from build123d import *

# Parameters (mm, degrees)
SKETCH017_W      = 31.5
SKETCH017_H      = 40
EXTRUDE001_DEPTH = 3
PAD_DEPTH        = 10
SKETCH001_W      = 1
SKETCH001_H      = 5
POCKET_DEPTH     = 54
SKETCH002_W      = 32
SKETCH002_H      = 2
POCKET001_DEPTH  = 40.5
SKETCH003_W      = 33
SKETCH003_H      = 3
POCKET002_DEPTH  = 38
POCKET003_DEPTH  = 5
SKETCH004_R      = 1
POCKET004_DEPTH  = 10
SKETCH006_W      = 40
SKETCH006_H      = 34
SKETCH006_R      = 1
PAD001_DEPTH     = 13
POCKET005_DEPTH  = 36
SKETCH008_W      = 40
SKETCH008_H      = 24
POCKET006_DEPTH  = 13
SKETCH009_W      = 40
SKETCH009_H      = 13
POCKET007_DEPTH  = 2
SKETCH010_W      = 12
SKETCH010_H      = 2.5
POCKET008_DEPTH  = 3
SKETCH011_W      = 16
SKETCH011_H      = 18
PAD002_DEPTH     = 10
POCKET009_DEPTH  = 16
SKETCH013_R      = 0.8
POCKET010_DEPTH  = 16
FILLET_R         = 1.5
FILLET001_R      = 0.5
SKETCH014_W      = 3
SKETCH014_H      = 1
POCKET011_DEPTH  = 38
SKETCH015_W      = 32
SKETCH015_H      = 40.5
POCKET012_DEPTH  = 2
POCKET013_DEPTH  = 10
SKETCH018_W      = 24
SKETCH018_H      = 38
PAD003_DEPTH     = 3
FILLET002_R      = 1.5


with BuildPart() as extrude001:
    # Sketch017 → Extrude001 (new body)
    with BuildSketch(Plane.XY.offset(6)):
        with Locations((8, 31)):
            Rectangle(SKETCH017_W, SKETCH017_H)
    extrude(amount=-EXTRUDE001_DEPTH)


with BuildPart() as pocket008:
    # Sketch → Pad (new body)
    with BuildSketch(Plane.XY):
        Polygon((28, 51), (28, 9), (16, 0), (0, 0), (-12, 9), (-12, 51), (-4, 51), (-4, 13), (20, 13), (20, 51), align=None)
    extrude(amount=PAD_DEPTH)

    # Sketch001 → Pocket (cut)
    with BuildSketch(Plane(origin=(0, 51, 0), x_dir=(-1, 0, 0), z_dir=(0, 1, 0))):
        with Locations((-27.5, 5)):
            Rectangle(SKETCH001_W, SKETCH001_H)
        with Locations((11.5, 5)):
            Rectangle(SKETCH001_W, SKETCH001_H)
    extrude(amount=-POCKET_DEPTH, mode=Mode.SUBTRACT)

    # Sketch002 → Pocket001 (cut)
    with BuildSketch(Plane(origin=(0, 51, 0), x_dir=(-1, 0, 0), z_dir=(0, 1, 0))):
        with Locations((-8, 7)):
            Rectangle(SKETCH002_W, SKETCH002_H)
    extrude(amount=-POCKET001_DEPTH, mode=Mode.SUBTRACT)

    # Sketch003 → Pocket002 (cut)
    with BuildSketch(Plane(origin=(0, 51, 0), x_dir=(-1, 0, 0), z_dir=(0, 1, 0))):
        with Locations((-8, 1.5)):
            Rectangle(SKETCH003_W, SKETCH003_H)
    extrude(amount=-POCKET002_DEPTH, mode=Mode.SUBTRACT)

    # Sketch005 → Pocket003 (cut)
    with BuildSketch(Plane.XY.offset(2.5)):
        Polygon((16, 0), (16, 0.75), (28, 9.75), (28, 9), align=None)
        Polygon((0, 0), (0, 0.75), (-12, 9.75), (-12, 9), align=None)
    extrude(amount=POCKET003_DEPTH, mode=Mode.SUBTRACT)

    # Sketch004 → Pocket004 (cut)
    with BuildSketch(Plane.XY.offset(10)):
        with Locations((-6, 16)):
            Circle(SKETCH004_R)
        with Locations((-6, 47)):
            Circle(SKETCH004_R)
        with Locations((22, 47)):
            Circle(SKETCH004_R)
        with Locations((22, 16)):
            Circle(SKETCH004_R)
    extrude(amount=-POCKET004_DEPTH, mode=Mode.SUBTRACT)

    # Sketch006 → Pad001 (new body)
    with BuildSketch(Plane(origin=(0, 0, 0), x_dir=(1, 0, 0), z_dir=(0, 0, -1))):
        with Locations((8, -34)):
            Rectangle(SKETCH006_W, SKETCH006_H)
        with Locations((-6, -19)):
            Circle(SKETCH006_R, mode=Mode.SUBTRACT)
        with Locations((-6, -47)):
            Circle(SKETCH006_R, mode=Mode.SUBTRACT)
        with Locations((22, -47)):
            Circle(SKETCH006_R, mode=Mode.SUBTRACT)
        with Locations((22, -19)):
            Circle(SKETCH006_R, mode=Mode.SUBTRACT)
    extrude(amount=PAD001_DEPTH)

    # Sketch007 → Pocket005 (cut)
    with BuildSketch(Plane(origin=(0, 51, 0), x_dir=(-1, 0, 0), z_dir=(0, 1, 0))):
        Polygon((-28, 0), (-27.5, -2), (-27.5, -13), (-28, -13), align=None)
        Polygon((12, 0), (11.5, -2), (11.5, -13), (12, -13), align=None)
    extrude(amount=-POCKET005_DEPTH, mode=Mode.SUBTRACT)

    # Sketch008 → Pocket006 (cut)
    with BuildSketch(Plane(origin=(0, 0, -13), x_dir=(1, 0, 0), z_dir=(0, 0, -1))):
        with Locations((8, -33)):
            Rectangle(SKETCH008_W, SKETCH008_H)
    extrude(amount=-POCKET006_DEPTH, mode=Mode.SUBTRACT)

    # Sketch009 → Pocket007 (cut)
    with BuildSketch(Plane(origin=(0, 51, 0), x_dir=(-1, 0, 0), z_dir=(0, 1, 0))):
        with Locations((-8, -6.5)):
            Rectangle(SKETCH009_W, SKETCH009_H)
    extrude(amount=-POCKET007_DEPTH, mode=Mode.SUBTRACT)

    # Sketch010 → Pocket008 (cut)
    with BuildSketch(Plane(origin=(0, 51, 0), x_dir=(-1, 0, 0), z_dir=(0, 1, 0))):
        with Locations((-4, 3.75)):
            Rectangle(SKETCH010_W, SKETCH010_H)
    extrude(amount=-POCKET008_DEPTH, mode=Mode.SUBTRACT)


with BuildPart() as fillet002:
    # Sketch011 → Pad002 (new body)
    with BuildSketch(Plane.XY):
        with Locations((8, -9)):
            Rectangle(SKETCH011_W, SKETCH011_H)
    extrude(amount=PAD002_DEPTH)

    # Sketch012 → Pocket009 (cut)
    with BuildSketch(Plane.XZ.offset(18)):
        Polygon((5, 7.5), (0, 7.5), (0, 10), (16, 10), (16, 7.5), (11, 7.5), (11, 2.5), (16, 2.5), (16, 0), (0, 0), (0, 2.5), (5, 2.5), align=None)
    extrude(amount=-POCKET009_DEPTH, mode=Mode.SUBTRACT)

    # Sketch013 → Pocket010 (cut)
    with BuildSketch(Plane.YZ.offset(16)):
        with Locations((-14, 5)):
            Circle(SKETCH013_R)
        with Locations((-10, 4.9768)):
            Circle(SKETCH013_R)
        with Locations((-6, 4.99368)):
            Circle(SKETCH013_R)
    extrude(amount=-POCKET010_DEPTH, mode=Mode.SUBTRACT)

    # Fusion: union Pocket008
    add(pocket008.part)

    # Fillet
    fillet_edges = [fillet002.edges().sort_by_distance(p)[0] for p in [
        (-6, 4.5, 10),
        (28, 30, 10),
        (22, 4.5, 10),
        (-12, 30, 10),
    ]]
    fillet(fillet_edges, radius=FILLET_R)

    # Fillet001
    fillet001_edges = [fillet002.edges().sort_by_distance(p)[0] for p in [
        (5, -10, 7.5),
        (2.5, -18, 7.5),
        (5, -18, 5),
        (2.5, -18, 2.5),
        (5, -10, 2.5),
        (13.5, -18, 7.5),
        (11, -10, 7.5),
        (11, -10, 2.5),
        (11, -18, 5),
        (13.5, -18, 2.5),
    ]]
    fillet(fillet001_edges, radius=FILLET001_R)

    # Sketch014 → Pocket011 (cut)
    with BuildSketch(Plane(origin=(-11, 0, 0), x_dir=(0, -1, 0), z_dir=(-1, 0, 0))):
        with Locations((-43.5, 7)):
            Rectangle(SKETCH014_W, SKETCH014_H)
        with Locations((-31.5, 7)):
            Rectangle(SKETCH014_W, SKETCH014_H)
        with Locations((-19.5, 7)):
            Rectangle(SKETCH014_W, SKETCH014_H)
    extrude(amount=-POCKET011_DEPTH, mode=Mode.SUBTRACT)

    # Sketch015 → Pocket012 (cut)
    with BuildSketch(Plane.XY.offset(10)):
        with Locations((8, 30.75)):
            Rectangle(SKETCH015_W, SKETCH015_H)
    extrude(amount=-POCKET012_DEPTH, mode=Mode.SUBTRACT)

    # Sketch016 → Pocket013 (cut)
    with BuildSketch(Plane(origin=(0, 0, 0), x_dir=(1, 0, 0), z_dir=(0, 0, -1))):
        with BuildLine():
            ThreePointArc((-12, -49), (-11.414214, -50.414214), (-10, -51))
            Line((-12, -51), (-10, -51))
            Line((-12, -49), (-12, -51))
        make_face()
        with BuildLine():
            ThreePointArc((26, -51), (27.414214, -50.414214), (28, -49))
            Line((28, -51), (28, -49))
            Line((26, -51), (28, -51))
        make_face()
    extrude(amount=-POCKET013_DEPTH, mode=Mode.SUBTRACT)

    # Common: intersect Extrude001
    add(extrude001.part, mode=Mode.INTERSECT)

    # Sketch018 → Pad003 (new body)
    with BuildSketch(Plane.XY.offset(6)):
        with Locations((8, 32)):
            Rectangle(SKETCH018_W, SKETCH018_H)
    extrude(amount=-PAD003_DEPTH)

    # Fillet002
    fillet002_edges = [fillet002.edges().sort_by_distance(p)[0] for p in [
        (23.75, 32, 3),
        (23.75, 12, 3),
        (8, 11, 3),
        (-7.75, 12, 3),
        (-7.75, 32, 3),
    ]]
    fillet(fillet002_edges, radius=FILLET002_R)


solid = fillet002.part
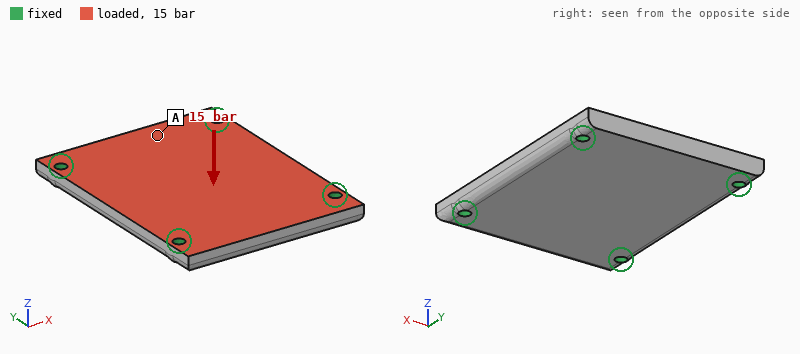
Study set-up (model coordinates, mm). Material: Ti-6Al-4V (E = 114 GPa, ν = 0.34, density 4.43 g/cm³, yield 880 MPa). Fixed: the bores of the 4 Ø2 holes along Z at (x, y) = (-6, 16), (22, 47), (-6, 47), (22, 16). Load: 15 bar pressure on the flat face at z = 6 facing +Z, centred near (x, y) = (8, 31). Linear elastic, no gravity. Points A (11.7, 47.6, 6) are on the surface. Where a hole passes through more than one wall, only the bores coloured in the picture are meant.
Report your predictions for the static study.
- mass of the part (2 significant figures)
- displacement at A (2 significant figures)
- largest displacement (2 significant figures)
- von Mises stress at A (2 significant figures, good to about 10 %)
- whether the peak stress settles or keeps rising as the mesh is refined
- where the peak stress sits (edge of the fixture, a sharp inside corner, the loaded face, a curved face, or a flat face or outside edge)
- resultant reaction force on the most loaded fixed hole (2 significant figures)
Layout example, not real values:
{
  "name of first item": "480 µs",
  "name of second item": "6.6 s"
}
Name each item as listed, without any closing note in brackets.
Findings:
{
  "mass of the part": "16 g",
  "displacement at A": "14 µm",
  "largest displacement": "35 µm",
  "von Mises stress at A": "36 MPa",
  "whether the peak stress settles or keeps rising as the mesh is refined": "keeps rising",
  "where the peak stress sits": "edge of the fixture",
  "resultant reaction force on the most loaded fixed hole": "480 N"
}
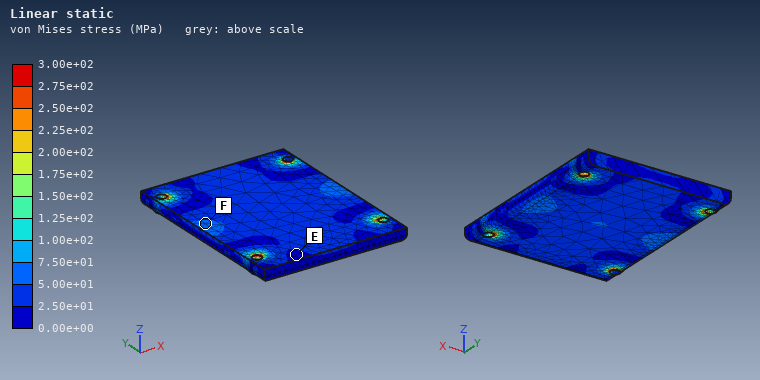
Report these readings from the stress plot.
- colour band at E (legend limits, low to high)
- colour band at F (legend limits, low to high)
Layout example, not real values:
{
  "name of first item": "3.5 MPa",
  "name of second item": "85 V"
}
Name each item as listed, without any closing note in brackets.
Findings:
{
  "colour band at E": "0.00e+00 to 2.50e+01 MPa",
  "colour band at F": "5.00e+01 to 7.50e+01 MPa"
}
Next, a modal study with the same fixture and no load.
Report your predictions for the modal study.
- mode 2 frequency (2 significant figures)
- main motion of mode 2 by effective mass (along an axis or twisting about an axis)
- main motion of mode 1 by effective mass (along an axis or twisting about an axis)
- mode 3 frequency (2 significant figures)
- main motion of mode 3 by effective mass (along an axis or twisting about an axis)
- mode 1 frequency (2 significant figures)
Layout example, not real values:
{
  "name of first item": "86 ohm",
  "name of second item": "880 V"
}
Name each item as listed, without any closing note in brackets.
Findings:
{
  "mode 2 frequency": "18 kHz",
  "main motion of mode 2 by effective mass": "twisting about Y",
  "main motion of mode 1 by effective mass": "along Z",
  "mode 3 frequency": "19 kHz",
  "main motion of mode 3 by effective mass": "twisting about X",
  "mode 1 frequency": "11 kHz"
}
